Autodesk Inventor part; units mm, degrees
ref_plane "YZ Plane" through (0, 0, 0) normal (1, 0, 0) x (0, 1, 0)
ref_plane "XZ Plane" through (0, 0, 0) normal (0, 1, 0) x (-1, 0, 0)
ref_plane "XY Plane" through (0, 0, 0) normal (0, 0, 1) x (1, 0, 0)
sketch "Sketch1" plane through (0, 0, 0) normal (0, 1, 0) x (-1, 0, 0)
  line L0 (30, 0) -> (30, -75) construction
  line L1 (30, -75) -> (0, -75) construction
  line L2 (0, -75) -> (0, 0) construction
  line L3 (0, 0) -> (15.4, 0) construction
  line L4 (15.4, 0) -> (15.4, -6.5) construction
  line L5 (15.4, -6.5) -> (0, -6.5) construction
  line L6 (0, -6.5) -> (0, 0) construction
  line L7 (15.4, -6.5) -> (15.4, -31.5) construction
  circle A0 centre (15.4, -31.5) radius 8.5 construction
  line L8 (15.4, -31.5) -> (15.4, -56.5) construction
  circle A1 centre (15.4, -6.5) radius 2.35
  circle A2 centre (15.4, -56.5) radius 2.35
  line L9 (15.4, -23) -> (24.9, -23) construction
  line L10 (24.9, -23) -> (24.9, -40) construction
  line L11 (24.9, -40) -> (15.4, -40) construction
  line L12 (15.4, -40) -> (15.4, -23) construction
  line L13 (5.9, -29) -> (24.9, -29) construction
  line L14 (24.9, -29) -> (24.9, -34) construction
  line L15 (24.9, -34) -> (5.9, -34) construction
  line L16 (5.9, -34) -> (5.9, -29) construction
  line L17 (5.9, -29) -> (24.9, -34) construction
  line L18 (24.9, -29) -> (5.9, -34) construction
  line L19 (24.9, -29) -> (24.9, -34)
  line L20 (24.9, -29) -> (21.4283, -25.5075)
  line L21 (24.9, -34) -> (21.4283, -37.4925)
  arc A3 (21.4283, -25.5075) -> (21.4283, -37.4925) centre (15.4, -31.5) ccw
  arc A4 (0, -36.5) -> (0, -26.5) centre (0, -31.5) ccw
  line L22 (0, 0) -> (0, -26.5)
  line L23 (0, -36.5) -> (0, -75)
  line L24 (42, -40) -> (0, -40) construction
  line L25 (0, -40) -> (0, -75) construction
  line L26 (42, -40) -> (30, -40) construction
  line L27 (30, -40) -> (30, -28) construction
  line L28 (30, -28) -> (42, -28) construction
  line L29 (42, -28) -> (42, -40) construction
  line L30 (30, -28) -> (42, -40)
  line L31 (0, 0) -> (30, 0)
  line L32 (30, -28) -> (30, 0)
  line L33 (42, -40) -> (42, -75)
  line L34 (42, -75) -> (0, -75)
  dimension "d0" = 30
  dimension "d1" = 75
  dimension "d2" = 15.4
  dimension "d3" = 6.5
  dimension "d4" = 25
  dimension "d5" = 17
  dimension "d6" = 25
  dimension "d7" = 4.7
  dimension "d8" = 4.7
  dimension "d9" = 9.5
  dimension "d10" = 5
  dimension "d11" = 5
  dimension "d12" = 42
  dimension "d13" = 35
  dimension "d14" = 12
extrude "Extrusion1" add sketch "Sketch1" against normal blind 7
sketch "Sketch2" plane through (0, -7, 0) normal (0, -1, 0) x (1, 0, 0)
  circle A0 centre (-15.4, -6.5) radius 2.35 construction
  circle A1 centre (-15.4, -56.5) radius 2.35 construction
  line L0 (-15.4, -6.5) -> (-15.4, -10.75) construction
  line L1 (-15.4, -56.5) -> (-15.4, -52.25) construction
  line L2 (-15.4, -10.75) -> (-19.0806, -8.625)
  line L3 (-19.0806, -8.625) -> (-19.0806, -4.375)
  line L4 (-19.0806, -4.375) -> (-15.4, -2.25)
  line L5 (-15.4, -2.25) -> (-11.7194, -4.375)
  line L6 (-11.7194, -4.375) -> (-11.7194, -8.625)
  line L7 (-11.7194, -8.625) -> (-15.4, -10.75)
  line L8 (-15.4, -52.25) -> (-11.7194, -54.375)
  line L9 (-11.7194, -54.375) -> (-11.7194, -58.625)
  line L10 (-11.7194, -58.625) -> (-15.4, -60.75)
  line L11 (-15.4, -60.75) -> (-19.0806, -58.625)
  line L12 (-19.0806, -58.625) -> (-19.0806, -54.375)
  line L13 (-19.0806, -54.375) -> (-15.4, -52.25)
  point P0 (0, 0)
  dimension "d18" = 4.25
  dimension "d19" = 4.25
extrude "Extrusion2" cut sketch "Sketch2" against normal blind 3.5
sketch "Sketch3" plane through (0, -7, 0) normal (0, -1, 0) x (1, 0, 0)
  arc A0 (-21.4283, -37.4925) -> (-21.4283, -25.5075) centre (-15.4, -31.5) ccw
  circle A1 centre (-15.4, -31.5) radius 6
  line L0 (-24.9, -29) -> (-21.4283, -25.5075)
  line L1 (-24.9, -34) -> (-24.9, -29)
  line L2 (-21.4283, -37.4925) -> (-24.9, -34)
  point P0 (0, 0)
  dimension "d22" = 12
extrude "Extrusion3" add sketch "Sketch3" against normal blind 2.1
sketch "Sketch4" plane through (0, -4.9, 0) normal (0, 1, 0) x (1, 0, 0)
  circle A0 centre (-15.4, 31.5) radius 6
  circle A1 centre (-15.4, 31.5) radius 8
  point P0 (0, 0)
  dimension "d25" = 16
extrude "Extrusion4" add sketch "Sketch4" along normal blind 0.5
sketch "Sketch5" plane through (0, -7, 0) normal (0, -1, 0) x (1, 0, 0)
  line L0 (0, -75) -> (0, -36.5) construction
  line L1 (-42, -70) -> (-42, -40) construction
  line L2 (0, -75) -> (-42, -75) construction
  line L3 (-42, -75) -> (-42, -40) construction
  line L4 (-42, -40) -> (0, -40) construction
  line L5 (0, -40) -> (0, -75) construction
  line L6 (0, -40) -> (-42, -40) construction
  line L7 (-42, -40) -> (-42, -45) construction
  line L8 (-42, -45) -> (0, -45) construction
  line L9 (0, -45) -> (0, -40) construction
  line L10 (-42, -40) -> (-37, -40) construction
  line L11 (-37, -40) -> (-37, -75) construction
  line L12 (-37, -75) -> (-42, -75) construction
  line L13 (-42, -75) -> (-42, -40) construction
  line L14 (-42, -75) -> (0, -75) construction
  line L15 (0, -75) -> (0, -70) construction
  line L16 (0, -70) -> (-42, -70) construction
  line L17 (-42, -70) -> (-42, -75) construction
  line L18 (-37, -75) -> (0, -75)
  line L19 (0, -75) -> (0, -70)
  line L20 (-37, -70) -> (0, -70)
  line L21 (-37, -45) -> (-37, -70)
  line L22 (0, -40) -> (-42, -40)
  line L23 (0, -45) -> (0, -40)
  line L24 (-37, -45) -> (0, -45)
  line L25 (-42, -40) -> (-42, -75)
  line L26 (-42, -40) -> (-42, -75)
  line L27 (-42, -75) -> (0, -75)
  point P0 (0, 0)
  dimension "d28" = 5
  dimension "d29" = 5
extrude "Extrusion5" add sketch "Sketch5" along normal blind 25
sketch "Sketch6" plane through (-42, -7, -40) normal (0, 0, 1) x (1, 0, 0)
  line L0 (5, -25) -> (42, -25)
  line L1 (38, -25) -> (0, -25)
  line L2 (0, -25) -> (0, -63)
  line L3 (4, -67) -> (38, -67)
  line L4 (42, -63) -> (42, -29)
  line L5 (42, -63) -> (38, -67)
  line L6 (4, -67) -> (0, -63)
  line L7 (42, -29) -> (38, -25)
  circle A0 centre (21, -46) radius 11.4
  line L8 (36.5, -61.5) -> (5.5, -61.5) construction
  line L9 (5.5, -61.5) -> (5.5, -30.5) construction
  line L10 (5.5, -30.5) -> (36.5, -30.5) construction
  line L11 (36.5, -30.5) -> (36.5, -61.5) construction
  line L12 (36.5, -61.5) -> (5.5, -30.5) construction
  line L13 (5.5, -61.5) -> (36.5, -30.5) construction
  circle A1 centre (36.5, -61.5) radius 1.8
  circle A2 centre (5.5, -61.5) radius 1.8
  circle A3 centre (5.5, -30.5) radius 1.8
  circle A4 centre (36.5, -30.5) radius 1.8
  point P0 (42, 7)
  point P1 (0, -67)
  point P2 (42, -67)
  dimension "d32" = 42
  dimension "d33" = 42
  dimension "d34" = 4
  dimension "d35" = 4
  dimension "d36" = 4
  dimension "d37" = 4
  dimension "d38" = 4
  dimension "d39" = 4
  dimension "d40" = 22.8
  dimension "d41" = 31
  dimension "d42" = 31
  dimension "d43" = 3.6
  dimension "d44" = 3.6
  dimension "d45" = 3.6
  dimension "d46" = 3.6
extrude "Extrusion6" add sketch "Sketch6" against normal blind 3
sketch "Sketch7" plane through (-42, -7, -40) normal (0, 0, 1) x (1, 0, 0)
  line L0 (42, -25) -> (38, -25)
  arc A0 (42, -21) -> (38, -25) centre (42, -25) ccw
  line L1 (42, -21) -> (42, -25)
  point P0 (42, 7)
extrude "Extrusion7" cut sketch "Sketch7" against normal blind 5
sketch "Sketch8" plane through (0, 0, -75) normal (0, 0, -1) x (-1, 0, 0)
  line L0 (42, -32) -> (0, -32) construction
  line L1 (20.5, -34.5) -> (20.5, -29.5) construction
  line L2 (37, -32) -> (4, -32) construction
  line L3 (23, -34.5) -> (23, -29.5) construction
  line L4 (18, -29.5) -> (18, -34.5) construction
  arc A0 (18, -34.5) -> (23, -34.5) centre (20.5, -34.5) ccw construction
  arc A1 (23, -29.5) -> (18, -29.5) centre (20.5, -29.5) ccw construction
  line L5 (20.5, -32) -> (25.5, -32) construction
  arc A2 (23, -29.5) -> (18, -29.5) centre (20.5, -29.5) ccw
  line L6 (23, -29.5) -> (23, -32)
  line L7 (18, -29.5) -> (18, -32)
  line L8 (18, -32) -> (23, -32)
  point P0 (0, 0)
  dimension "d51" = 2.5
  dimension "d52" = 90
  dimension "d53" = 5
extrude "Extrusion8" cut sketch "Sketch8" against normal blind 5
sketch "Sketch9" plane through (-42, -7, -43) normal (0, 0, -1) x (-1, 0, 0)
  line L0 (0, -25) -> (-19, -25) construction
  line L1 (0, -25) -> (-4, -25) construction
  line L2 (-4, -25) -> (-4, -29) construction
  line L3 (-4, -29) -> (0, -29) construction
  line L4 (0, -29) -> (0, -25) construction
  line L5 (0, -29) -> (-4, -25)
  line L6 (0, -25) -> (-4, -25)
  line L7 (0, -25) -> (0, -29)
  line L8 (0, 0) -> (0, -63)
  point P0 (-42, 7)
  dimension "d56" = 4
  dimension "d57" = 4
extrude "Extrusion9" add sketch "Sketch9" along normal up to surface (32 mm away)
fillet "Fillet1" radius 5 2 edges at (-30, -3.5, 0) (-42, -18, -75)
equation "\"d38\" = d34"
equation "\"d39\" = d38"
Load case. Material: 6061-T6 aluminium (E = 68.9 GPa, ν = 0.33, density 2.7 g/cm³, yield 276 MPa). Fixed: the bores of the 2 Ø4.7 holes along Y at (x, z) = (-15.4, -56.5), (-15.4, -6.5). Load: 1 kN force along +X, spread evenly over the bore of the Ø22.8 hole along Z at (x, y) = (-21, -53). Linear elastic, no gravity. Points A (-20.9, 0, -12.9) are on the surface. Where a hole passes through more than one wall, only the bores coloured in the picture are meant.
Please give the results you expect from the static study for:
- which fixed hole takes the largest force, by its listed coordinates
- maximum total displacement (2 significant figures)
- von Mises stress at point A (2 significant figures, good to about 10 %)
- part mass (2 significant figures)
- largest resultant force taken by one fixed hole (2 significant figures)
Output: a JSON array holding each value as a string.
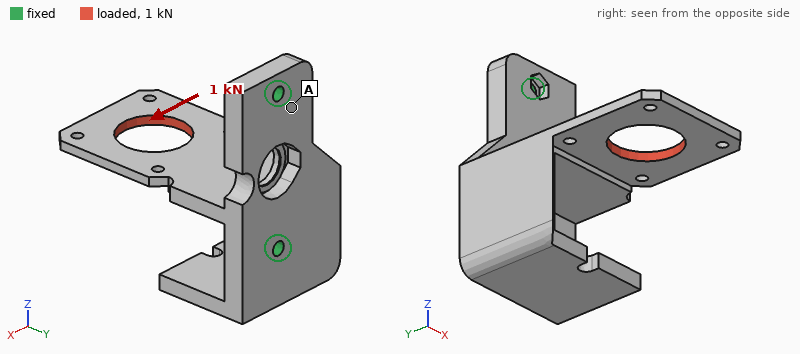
["(-15.4, -56.5)", "0.90 mm", "54 MPa", "93 g", "660 N"]
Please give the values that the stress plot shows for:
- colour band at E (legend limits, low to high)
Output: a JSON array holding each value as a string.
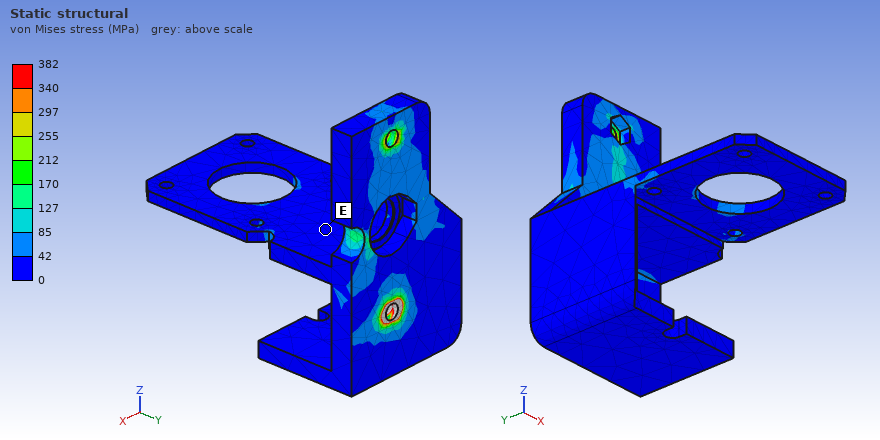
["0 to 42 MPa"]
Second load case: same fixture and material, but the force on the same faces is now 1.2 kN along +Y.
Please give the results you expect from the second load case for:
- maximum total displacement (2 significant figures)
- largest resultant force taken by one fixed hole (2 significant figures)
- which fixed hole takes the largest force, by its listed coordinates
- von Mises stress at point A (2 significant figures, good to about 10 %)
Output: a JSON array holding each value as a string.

["0.16 mm", "1.1 kN", "(-15.4, -56.5)", "16 MPa"]
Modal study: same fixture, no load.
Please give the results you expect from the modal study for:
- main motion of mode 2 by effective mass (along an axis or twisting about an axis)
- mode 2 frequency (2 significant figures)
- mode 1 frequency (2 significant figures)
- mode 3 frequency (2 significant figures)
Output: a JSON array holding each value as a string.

["along X", "1400 Hz", "1000 Hz", "2500 Hz"]
